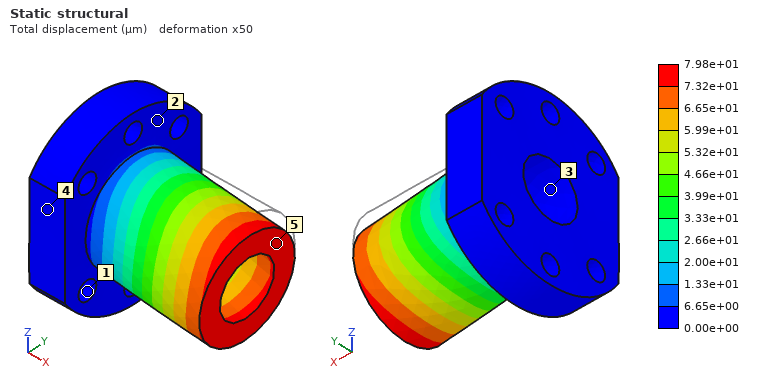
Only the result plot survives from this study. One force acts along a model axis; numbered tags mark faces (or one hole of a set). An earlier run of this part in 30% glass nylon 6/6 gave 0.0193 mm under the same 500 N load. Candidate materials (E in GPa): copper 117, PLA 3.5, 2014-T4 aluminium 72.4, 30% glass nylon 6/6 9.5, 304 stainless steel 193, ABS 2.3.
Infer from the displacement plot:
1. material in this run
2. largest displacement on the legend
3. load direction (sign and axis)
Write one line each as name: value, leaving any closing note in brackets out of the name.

material in this run: ABS
largest displacement on the legend: 7.98e+01 µm
load direction: -Z
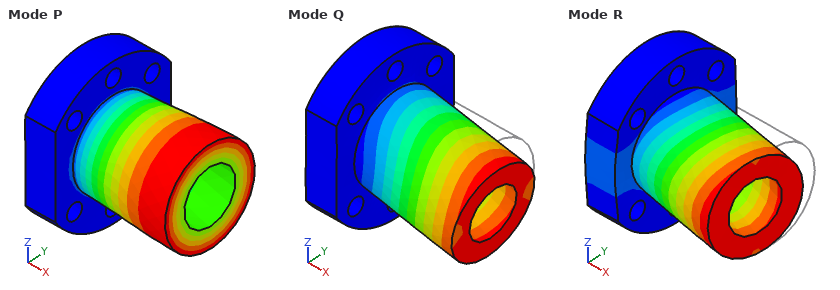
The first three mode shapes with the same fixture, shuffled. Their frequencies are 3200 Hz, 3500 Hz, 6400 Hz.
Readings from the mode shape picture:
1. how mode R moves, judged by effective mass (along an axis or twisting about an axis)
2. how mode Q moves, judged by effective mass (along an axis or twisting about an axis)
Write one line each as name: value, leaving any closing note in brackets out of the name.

how mode R moves, judged by effective mass: along Y
how mode Q moves, judged by effective mass: along Z
